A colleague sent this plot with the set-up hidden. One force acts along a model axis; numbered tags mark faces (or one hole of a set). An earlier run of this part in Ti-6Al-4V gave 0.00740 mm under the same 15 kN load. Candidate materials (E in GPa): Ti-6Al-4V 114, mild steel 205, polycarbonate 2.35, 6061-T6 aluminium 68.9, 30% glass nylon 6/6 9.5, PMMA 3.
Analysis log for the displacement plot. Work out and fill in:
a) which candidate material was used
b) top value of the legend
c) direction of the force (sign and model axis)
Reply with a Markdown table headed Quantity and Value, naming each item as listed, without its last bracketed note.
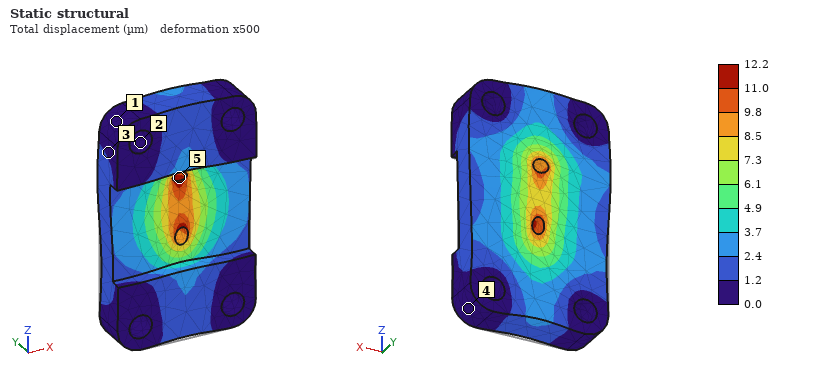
| Quantity | Value |
|---|---|
| which candidate material was used | 6061-T6 aluminium |
| top value of the legend | 12.2 µm |
| direction of the force | +Z |
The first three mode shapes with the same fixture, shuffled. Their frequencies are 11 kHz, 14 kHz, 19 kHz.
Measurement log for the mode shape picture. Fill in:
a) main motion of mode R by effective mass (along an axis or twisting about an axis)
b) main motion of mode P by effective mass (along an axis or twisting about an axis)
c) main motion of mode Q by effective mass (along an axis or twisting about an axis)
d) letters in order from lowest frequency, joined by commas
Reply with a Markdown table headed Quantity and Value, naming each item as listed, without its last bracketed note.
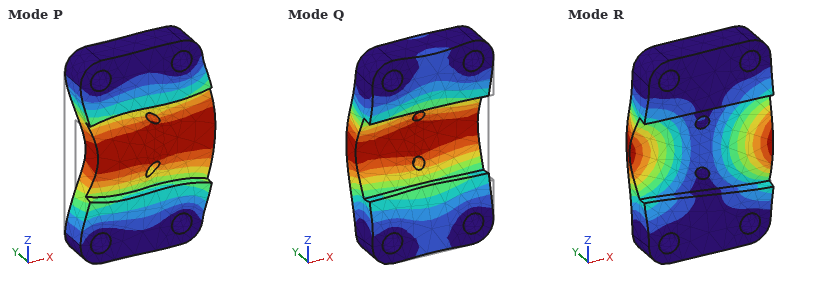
| Quantity | Value |
|---|---|
| main motion of mode R by effective mass | twisting about Z |
| main motion of mode P by effective mass | along X |
| main motion of mode Q by effective mass | along Y |
| letters in order from lowest frequency, joined by commas | Q, R, P |
